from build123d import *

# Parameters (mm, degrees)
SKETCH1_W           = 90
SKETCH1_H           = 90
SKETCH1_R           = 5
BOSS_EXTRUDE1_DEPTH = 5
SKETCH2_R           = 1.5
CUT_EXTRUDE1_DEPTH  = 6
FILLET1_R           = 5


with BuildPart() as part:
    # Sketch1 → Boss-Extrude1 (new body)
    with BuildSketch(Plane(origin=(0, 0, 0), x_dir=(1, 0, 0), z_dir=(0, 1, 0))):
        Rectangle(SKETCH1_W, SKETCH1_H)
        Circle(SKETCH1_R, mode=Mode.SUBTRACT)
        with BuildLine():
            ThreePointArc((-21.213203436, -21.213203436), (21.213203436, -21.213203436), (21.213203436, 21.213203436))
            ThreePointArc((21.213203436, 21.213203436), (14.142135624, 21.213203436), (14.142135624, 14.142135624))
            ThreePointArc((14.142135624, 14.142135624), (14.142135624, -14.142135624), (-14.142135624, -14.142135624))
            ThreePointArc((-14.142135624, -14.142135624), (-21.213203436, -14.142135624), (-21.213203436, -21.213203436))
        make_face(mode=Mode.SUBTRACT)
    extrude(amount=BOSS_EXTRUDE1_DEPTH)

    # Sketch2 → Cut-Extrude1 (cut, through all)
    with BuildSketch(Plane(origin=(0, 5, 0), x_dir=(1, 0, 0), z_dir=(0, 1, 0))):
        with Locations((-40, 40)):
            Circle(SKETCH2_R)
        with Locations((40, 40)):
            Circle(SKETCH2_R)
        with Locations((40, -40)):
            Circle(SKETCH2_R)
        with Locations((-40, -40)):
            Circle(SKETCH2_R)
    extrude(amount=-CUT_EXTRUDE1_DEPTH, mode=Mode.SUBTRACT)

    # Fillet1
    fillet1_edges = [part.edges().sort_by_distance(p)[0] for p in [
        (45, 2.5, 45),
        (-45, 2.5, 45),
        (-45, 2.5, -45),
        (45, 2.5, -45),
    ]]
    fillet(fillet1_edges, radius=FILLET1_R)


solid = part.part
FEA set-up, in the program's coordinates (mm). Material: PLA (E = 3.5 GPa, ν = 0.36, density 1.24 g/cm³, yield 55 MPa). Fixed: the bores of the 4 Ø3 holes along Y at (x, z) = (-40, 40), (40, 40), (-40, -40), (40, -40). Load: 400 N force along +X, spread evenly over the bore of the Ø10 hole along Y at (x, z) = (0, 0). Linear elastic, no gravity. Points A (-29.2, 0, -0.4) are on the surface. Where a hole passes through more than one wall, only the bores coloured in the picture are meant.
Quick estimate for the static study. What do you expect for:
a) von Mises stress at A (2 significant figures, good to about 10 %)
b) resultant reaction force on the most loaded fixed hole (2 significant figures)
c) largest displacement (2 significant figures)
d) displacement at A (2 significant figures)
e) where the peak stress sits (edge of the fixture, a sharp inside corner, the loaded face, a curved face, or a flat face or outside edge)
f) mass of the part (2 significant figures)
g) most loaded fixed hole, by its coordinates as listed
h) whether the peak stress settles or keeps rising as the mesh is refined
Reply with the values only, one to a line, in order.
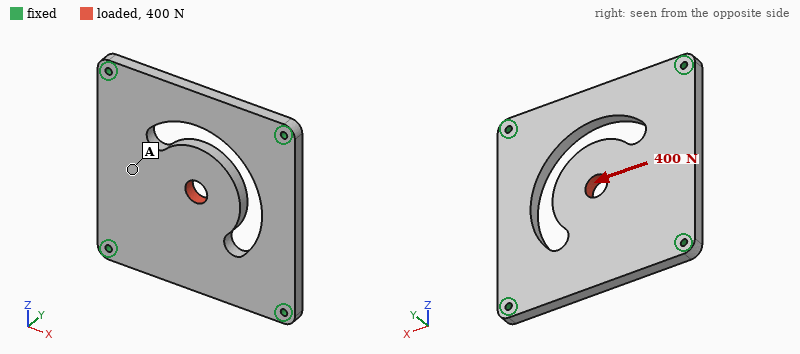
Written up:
1.3 MPa
190 N
84 µm
50 µm
edge of the fixture
44 g
(-40, -40)
keeps rising
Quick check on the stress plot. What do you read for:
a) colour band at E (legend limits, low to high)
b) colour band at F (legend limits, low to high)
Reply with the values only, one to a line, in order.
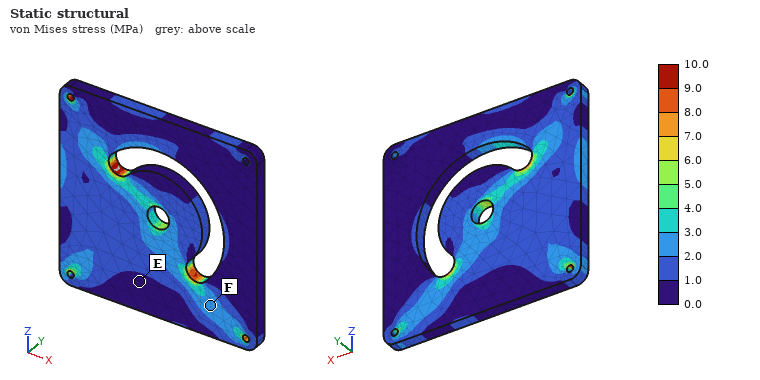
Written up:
0.0 to 1.0 MPa
2.0 to 3.0 MPa
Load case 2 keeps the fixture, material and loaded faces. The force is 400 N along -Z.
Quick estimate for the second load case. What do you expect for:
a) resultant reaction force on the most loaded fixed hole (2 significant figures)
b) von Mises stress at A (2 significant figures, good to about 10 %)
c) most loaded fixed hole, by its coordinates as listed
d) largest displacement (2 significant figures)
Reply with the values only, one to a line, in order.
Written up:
190 N
0.96 MPa
(-40, -40)
84 µm
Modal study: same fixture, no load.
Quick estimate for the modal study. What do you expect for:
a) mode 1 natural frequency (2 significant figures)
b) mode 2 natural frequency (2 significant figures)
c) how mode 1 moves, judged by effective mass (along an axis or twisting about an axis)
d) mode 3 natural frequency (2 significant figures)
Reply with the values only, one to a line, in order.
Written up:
570 Hz
1300 Hz
along Y
1300 Hz
